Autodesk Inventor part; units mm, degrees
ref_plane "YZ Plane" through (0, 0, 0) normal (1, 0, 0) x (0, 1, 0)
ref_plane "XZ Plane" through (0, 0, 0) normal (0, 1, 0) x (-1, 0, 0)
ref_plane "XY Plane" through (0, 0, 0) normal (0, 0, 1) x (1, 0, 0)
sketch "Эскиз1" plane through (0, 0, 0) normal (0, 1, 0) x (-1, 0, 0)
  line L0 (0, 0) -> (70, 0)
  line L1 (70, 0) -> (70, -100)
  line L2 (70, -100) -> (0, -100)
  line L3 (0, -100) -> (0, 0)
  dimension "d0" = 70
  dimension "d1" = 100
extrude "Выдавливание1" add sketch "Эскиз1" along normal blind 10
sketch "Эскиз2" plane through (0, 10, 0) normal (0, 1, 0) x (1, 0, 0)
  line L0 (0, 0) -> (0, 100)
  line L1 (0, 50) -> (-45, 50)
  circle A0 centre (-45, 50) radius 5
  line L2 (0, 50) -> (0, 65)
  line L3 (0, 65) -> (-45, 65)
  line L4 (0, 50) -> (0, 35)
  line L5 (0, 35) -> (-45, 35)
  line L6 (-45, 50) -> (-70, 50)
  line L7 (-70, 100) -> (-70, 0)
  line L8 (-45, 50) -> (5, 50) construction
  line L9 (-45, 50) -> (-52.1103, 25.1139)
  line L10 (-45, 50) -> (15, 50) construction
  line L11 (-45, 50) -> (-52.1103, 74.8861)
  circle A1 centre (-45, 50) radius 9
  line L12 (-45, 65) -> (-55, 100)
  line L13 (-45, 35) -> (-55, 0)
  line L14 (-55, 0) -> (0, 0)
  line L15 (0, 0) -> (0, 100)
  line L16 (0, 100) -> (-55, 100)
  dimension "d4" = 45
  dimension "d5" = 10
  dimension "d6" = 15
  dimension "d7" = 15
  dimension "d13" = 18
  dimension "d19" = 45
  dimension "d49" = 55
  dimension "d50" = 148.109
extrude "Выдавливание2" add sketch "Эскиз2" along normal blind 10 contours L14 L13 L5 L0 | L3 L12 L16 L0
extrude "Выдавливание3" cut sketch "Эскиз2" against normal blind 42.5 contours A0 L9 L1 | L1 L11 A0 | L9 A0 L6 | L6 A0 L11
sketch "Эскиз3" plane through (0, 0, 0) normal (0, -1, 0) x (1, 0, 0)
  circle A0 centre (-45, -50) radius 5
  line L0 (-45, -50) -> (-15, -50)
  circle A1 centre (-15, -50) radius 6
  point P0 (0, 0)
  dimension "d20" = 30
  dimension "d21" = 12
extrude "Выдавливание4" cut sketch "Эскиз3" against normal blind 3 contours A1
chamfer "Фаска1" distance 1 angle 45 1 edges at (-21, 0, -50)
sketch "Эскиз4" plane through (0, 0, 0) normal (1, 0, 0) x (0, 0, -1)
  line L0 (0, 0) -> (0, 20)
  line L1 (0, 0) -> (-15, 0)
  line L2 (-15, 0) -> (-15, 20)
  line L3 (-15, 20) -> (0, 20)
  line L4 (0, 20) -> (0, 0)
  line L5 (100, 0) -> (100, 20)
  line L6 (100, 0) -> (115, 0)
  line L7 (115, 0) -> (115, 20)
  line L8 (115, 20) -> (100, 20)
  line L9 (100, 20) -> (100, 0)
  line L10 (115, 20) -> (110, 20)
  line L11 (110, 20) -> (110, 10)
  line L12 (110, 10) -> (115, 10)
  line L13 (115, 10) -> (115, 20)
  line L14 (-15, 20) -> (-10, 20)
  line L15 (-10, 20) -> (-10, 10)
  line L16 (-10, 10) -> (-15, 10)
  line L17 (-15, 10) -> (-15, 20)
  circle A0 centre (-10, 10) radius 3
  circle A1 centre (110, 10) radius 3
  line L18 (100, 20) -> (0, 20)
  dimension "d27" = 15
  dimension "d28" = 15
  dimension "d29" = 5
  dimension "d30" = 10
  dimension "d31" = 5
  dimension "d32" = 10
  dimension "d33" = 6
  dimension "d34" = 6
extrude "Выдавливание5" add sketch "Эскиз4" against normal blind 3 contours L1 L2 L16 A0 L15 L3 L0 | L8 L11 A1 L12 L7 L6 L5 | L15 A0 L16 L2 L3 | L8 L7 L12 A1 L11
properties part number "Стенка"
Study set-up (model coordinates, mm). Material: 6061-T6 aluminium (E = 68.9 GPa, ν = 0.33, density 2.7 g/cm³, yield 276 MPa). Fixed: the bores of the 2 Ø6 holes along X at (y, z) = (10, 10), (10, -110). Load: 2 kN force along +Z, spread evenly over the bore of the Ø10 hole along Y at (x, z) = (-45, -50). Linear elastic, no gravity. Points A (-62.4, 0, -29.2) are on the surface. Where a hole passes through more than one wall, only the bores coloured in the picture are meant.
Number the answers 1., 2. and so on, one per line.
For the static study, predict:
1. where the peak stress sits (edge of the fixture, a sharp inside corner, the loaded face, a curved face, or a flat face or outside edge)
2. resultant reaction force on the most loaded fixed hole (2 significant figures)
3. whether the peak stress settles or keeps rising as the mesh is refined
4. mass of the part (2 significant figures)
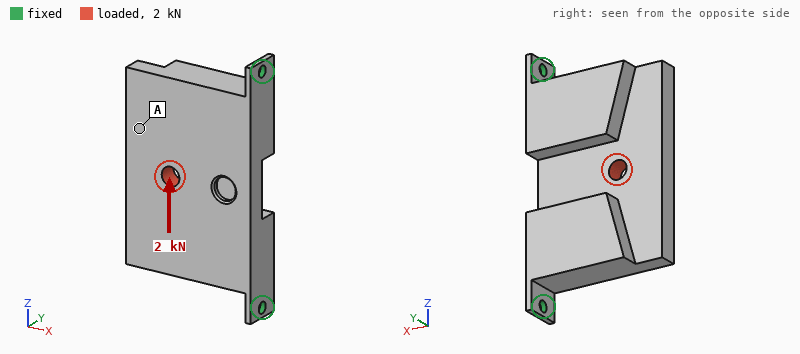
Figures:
1. edge of the fixture
2. 1.3 kN
3. keeps rising
4. 280 g
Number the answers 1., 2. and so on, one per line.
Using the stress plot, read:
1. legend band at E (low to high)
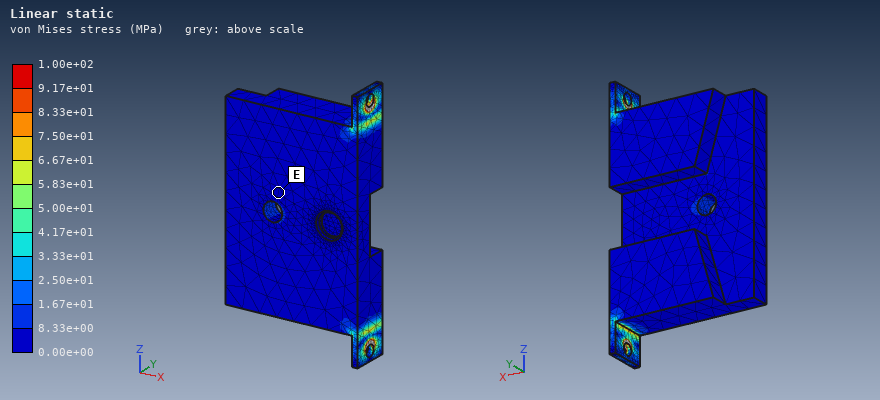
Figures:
1. 0.00e+00 to 8.33e+00 MPa
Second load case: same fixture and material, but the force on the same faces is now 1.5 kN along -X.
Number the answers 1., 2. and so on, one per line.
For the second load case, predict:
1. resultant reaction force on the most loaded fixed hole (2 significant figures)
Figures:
1. 890 N
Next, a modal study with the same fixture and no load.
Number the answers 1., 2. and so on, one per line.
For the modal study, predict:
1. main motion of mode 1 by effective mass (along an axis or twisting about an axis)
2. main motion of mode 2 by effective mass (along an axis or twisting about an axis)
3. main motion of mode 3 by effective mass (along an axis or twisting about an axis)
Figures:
1. along Y
2. along X
3. along Z
